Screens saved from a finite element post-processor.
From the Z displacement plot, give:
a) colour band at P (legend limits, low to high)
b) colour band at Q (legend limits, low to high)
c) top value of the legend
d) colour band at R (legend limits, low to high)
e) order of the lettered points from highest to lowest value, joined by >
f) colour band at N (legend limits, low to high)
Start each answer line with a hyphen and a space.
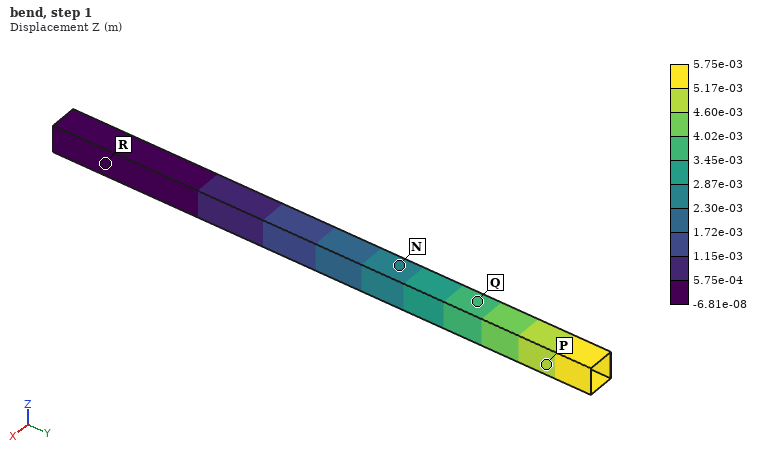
- 4.60e-03 to 5.17e-03 m
- 3.45e-03 to 4.02e-03 m
- 5.75e-03 m
- -6.81e-08 to 5.75e-04 m
- P > Q > N > R
- 2.30e-03 to 2.87e-03 m
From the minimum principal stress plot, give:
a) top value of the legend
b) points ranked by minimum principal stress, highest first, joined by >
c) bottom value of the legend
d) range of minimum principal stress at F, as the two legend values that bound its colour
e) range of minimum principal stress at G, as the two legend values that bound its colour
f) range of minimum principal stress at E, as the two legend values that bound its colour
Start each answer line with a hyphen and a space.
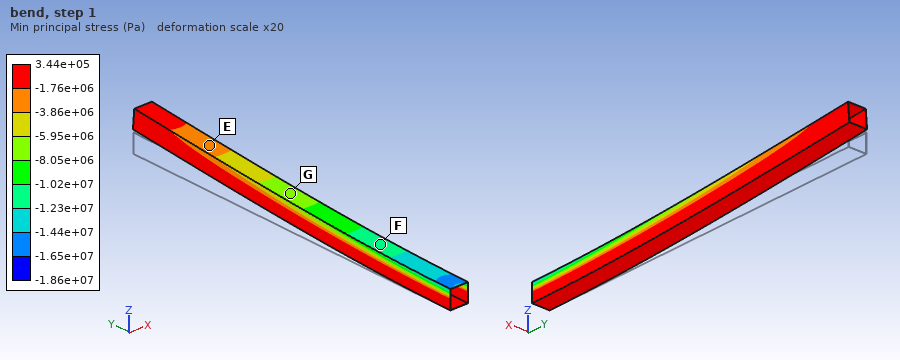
- 3.44e+05 Pa
- E > G > F
- -1.86e+07 Pa
- -1.23e+07 to -1.02e+07 Pa
- -8.05e+06 to -5.95e+06 Pa
- -3.86e+06 to -1.76e+06 Pa
